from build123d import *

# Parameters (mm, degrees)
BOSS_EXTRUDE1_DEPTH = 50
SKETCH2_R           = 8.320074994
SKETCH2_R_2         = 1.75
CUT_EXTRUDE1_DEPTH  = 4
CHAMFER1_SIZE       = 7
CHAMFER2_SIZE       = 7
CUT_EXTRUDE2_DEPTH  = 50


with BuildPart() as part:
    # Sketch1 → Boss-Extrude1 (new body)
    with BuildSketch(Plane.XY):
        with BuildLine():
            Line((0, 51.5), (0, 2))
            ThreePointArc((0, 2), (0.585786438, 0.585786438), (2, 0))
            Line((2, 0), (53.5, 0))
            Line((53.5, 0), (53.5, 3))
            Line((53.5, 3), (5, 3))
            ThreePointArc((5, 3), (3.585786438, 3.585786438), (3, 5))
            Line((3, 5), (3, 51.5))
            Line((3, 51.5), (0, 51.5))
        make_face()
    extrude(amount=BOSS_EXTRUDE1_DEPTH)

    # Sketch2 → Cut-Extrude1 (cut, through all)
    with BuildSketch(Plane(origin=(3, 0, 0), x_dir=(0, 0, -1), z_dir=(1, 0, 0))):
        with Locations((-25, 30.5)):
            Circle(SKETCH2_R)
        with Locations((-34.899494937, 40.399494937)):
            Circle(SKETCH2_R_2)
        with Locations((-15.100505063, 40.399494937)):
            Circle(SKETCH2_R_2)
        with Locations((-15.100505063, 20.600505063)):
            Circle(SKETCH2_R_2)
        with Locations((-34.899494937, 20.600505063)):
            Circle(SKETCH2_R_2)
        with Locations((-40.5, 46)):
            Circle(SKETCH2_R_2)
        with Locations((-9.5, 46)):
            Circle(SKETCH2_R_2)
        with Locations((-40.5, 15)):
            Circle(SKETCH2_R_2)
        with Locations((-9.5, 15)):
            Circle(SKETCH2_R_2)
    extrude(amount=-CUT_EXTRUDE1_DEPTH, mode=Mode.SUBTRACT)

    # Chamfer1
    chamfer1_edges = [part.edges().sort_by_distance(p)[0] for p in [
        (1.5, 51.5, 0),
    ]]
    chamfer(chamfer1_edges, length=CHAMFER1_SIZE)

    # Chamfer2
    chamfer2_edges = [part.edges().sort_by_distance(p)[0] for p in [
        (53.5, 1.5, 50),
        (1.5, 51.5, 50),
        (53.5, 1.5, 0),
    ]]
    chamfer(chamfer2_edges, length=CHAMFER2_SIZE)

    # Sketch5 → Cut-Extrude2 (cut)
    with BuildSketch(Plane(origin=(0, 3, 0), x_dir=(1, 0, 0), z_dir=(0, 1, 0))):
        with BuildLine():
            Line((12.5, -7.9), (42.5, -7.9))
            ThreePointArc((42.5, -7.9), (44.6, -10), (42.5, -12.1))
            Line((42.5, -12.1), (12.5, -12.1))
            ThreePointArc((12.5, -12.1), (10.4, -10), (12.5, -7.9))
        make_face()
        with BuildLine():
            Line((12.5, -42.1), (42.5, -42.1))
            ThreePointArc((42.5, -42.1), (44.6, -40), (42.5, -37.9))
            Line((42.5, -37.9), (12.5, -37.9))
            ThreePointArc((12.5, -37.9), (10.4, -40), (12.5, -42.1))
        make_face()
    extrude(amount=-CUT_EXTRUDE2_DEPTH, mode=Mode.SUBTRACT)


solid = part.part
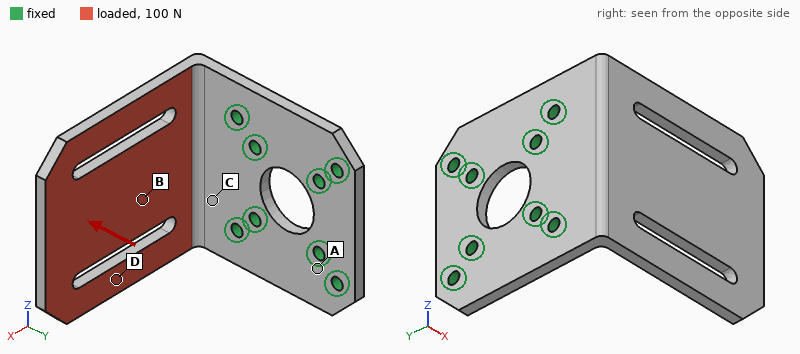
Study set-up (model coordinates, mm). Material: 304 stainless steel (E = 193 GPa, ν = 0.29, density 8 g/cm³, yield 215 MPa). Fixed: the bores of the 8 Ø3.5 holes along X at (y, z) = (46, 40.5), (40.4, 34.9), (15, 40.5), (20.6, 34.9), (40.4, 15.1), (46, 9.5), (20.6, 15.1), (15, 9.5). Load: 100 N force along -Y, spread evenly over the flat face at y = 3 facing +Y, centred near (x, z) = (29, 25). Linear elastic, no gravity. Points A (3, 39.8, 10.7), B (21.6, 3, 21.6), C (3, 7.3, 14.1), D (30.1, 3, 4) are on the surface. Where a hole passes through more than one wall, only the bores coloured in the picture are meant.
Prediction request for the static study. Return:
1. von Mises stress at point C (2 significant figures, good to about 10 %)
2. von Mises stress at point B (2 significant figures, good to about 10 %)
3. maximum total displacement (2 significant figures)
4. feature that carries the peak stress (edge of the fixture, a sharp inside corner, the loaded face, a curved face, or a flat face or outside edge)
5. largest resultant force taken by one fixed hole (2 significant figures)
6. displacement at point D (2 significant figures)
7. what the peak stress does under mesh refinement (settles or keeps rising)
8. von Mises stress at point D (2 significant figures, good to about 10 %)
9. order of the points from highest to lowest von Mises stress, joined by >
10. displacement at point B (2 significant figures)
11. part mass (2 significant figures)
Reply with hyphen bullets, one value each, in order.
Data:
- 34 MPa
- 16 MPa
- 0.16 mm
- edge of the fixture
- 70 N
- 0.075 mm
- keeps rising
- 8.9 MPa
- C > B > D > A
- 0.048 mm
- 110 g
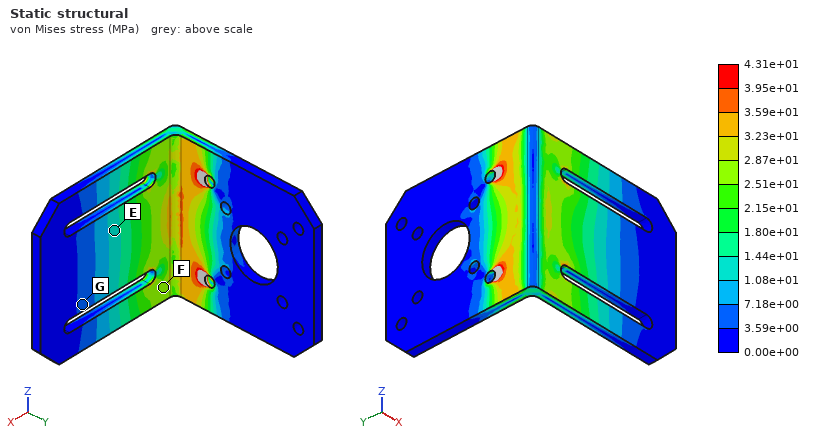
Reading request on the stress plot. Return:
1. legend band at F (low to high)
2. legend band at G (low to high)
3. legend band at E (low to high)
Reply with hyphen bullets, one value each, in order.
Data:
- 2.51e+01 to 2.87e+01 MPa
- 3.59e+00 to 7.18e+00 MPa
- 1.08e+01 to 1.44e+01 MPa
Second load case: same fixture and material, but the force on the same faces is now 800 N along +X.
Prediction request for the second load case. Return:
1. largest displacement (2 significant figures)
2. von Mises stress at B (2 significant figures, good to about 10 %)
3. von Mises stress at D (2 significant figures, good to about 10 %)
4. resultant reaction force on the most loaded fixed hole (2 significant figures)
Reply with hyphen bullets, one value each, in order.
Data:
- 98 µm
- 15 MPa
- 13 MPa
- 520 N
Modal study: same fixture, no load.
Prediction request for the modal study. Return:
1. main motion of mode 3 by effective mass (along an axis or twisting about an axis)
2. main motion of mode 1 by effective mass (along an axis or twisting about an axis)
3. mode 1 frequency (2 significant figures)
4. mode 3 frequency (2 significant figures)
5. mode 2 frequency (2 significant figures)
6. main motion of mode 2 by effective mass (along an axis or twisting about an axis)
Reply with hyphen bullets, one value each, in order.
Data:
- along Z
- along Y
- 680 Hz
- 2600 Hz
- 1800 Hz
- along Z
